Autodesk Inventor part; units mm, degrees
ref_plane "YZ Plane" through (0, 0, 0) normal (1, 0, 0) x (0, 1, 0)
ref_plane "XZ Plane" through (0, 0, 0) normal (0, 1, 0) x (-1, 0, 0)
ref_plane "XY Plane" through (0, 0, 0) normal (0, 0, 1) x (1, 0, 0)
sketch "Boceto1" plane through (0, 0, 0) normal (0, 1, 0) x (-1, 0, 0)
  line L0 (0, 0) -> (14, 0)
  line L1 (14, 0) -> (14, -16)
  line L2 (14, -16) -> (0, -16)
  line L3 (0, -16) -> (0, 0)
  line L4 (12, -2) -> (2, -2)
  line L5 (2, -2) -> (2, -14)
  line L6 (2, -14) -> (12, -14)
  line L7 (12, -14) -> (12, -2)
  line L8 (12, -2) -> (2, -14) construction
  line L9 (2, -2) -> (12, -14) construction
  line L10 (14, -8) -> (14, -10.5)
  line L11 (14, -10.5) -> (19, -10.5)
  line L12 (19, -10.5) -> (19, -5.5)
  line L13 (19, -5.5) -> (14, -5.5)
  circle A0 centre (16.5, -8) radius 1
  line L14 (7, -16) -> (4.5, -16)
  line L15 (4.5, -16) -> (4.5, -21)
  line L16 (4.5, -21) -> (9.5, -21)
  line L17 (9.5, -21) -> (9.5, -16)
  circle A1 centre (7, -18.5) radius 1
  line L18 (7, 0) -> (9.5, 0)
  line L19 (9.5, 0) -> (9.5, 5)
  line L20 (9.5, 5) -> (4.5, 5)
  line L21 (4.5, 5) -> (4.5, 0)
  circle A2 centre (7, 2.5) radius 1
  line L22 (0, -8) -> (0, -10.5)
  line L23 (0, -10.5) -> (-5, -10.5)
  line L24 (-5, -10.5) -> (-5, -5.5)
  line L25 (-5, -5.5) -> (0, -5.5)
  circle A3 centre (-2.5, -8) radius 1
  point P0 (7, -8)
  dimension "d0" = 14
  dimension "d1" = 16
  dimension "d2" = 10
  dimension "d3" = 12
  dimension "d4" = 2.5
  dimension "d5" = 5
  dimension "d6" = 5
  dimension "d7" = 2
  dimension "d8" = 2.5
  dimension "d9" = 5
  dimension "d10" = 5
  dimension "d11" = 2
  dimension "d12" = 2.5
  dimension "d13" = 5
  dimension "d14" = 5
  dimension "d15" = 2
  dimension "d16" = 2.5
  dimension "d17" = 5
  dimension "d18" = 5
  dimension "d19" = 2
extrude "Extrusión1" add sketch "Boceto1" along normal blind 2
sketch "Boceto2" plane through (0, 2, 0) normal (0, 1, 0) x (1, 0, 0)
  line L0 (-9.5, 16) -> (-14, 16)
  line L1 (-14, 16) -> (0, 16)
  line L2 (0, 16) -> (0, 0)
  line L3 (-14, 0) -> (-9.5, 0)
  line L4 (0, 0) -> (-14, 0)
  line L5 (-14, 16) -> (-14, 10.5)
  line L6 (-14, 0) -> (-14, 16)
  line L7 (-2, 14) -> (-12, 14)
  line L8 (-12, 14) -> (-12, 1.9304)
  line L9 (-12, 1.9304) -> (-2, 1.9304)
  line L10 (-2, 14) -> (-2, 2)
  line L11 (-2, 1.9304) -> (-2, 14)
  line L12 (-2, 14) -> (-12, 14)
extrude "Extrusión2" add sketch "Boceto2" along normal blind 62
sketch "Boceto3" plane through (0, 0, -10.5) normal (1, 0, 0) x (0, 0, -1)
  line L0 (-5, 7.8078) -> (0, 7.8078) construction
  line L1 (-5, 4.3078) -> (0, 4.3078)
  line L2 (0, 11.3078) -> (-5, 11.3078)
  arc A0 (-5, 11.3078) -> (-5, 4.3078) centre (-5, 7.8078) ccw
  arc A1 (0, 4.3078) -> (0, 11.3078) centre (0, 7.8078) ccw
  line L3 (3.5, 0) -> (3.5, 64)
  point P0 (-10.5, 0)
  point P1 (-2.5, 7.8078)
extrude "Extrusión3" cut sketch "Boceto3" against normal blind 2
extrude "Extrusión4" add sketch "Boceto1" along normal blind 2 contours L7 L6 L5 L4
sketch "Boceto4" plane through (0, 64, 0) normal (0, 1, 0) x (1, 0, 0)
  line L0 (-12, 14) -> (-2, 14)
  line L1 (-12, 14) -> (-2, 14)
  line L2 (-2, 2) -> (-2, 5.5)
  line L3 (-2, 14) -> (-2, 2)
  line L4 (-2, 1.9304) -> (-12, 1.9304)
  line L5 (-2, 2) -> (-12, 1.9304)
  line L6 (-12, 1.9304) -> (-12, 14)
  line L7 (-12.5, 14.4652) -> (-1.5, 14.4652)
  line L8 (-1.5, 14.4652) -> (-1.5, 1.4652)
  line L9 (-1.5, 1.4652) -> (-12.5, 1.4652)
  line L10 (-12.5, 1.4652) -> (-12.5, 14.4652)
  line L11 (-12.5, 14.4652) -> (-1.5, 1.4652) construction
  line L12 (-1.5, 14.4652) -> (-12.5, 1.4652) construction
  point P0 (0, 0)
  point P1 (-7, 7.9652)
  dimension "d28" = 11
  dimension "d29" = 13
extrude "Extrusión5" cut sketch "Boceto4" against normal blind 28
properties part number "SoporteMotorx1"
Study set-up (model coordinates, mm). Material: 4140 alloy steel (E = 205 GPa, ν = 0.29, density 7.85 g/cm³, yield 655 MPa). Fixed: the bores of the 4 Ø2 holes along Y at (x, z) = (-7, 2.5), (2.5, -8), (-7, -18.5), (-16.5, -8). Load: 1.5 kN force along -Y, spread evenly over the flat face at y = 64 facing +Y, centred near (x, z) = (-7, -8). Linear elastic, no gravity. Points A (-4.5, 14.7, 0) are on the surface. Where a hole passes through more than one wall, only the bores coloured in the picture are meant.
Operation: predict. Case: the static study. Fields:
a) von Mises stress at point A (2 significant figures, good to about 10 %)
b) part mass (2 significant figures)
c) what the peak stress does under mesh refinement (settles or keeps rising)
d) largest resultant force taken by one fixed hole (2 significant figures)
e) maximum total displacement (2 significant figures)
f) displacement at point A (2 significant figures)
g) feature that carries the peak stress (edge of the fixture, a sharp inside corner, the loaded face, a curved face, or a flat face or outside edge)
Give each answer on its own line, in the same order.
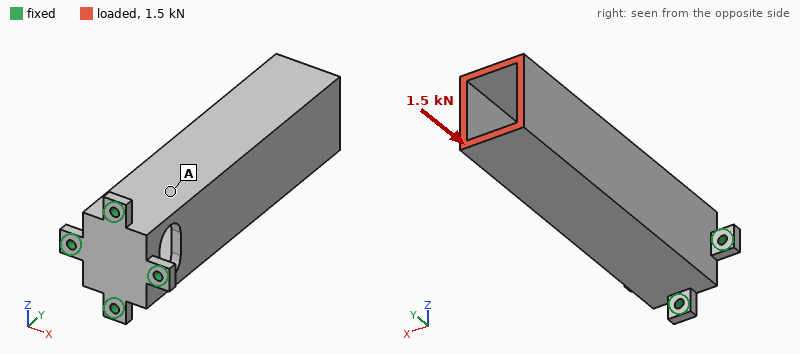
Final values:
24 MPa
49 g
keeps rising
470 N
18 µm
5.7 µm
edge of the fixture
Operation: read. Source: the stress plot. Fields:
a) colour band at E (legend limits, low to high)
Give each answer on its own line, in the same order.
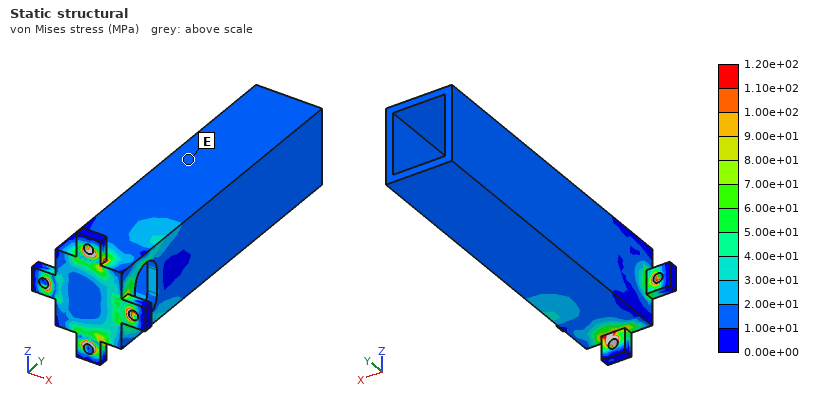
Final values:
1.00e+01 to 2.00e+01 MPa
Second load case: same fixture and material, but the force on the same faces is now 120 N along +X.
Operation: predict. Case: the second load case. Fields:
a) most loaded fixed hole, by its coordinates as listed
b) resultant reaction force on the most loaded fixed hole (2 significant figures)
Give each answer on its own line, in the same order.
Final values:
(-16.5, -8)
560 N
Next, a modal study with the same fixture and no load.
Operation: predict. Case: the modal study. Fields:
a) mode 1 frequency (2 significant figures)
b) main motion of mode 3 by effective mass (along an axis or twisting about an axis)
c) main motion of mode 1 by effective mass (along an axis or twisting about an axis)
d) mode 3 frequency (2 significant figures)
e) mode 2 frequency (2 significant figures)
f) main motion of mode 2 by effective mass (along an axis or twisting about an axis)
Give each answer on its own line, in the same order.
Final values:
1800 Hz
twisting about Y
along X
8800 Hz
2400 Hz
along Z
